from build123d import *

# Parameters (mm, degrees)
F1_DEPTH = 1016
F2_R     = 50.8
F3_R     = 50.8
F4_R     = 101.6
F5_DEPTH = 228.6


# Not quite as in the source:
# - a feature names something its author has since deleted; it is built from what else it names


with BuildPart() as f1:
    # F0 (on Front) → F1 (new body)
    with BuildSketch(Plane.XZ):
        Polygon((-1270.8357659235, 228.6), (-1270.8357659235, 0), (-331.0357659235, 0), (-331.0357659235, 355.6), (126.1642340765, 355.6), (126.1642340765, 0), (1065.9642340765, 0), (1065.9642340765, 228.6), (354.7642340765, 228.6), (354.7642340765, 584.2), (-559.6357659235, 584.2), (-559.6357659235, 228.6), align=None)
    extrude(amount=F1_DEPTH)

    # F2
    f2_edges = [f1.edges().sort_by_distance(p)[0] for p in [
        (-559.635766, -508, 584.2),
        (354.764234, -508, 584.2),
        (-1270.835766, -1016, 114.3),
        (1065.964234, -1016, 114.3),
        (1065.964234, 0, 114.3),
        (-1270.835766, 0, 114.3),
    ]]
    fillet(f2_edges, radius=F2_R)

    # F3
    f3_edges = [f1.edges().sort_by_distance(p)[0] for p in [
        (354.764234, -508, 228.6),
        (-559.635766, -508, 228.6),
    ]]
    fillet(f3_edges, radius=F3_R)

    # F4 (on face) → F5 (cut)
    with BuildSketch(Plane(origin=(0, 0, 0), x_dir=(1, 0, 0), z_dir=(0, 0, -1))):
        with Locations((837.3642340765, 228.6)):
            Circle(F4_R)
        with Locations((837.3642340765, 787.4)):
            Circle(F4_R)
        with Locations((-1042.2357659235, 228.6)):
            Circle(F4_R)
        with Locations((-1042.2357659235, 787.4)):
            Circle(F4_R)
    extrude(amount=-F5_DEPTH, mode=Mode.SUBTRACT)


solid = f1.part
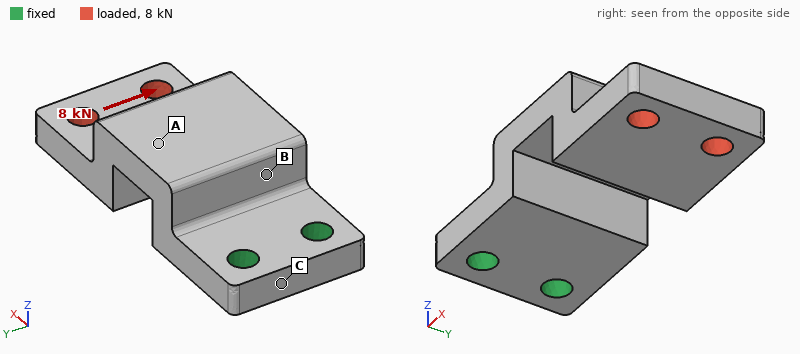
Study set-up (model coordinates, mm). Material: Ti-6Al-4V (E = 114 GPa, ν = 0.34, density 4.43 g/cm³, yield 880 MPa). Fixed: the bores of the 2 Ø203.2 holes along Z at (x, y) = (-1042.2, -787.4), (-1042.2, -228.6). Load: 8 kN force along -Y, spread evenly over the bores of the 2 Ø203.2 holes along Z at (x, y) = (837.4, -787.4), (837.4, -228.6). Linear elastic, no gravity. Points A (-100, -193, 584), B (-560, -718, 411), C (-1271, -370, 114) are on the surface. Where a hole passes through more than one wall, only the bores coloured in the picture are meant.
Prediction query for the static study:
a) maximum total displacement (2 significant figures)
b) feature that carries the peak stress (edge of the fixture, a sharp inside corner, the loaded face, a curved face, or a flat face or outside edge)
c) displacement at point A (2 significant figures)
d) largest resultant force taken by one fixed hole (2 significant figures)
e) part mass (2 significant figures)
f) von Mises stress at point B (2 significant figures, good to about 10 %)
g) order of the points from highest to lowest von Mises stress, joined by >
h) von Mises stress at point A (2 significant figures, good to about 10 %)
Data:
35 µm
a curved face
7.4 µm
22 kN
3000 kg
0.47 MPa
B > A > C
0.21 MPa
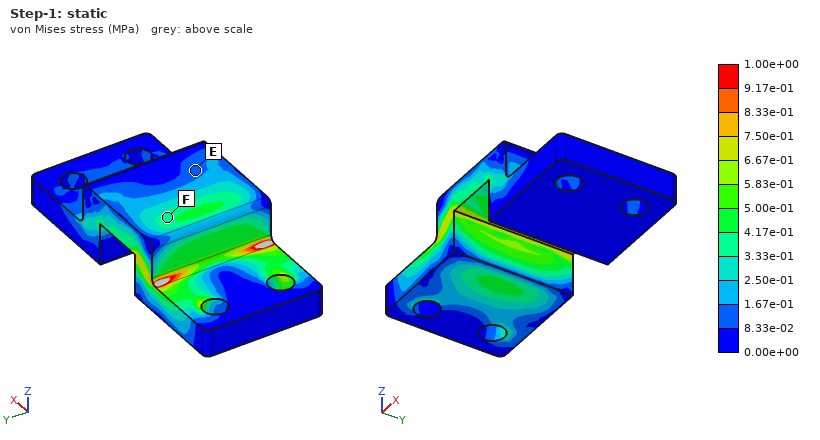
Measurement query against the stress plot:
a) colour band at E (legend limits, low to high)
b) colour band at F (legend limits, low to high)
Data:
8.33e-02 to 1.67e-01 MPa
3.33e-01 to 4.17e-01 MPa
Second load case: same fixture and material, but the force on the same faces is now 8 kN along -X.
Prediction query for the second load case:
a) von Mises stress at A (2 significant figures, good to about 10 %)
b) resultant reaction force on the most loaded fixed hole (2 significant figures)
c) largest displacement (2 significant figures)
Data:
0.27 MPa
4.0 kN
26 µm
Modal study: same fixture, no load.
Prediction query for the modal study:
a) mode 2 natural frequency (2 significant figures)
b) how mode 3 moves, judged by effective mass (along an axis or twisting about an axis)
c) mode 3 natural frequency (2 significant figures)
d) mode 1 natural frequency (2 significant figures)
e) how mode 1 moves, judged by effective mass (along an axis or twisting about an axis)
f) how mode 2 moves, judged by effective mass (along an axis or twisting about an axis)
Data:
93 Hz
along X
150 Hz
40 Hz
along Z
along Y
